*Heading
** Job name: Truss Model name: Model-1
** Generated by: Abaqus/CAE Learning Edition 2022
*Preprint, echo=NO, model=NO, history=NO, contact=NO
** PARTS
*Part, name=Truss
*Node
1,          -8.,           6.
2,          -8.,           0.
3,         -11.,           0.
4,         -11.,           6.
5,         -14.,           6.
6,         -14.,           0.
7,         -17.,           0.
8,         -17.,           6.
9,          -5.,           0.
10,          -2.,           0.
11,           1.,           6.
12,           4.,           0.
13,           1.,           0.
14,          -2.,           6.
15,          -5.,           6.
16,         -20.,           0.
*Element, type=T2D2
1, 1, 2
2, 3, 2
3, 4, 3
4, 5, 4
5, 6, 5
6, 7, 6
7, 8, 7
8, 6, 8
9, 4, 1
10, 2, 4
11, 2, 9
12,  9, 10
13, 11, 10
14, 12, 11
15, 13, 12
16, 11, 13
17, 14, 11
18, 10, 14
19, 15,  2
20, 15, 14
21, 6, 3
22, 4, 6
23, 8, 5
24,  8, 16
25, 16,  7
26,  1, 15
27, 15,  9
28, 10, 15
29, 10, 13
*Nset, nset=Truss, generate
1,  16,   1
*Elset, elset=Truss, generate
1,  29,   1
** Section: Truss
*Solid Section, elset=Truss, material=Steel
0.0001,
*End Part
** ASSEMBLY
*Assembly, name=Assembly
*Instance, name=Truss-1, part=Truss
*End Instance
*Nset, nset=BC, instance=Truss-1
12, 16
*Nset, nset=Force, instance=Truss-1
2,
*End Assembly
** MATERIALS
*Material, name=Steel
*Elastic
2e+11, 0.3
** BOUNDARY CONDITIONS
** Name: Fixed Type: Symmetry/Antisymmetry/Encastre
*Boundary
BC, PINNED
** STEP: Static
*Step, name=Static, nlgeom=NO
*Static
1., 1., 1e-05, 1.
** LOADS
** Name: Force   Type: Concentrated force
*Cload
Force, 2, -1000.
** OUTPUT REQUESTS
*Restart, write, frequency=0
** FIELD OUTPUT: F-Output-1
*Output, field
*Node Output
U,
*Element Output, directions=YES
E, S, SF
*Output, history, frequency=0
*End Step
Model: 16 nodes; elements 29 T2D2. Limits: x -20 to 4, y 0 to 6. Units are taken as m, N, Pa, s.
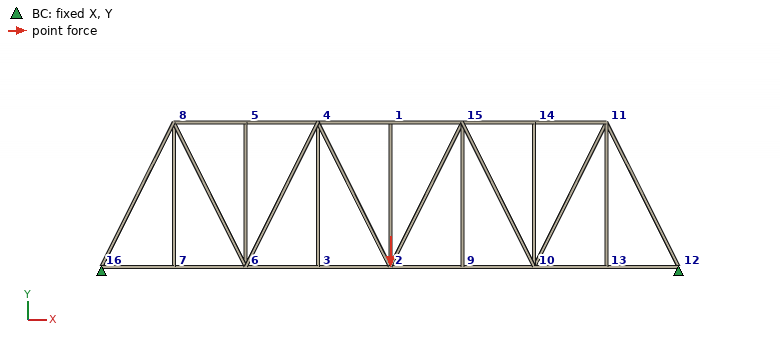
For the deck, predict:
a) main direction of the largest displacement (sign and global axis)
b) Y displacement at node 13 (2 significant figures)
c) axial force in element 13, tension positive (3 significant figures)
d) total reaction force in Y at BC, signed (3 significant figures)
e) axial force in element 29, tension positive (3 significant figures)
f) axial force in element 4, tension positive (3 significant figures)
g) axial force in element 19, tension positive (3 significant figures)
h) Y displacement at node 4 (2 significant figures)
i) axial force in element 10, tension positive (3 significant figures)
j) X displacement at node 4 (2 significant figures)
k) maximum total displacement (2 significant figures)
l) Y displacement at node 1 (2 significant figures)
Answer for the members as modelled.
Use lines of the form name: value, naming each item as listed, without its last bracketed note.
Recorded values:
main direction of the largest displacement: -Y
Y displacement at node 13: -3.6e-04 m
axial force in element 13, tension positive: 559 N
total reaction force in Y at BC, signed: 1000 N
axial force in element 29, tension positive: -250 N
axial force in element 4, tension positive: -500 N
axial force in element 19, tension positive: 559 N
Y displacement at node 4: -0.0011 m
axial force in element 10, tension positive: 559 N
X displacement at node 4: 1.5e-04 m
maximum total displacement: 0.0014 m
Y displacement at node 1: -0.0014 m
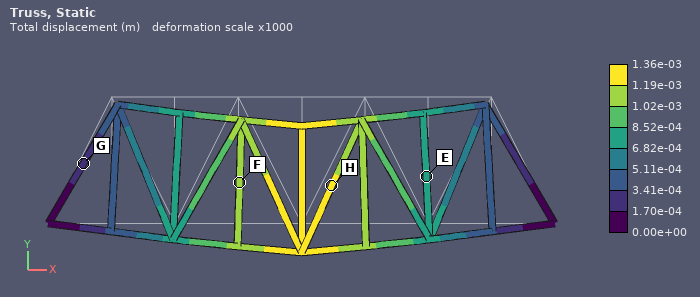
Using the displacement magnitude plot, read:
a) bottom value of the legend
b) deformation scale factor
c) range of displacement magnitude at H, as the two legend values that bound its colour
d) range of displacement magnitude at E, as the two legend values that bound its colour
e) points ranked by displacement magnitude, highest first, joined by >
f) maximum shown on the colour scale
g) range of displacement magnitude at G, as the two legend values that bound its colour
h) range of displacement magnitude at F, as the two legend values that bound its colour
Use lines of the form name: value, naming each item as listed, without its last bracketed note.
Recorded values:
bottom value of the legend: 0.00e+00 m
deformation scale factor: 1000
range of displacement magnitude at H, as the two legend values that bound its colour: 1.19e-03 to 1.36e-03 m
range of displacement magnitude at E, as the two legend values that bound its colour: 6.82e-04 to 8.52e-04 m
points ranked by displacement magnitude, highest first, joined by >: H > F > E > G
maximum shown on the colour scale: 1.36e-03 m
range of displacement magnitude at G, as the two legend values that bound its colour: 1.70e-04 to 3.41e-04 m
range of displacement magnitude at F, as the two legend values that bound its colour: 1.02e-03 to 1.19e-03 m
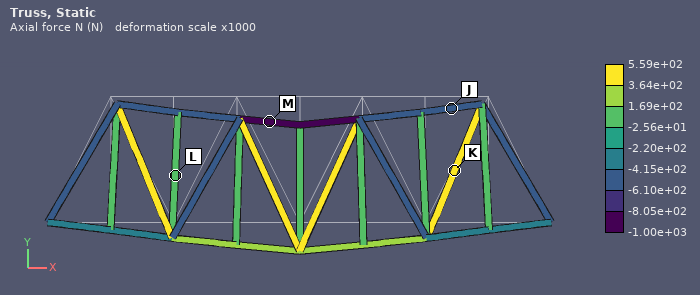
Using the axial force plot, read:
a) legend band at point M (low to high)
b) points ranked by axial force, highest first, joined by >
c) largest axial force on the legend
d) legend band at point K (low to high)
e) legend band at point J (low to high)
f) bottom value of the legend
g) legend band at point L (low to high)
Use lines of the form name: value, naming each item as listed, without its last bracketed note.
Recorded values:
legend band at point M: -1.00e+03 to -8.05e+02 N
points ranked by axial force, highest first, joined by >: K > L > J > M
largest axial force on the legend: 5.59e+02 N
legend band at point K: 3.64e+02 to 5.59e+02 N
legend band at point J: -6.10e+02 to -4.15e+02 N
bottom value of the legend: -1.00e+03 N
legend band at point L: -2.56e+01 to 1.69e+02 N
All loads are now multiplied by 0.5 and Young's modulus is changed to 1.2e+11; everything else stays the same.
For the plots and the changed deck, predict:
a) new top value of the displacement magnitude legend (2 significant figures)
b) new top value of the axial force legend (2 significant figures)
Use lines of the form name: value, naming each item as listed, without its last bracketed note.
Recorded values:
new top value of the displacement magnitude legend: 0.0011 m
new top value of the axial force legend: 280 N
